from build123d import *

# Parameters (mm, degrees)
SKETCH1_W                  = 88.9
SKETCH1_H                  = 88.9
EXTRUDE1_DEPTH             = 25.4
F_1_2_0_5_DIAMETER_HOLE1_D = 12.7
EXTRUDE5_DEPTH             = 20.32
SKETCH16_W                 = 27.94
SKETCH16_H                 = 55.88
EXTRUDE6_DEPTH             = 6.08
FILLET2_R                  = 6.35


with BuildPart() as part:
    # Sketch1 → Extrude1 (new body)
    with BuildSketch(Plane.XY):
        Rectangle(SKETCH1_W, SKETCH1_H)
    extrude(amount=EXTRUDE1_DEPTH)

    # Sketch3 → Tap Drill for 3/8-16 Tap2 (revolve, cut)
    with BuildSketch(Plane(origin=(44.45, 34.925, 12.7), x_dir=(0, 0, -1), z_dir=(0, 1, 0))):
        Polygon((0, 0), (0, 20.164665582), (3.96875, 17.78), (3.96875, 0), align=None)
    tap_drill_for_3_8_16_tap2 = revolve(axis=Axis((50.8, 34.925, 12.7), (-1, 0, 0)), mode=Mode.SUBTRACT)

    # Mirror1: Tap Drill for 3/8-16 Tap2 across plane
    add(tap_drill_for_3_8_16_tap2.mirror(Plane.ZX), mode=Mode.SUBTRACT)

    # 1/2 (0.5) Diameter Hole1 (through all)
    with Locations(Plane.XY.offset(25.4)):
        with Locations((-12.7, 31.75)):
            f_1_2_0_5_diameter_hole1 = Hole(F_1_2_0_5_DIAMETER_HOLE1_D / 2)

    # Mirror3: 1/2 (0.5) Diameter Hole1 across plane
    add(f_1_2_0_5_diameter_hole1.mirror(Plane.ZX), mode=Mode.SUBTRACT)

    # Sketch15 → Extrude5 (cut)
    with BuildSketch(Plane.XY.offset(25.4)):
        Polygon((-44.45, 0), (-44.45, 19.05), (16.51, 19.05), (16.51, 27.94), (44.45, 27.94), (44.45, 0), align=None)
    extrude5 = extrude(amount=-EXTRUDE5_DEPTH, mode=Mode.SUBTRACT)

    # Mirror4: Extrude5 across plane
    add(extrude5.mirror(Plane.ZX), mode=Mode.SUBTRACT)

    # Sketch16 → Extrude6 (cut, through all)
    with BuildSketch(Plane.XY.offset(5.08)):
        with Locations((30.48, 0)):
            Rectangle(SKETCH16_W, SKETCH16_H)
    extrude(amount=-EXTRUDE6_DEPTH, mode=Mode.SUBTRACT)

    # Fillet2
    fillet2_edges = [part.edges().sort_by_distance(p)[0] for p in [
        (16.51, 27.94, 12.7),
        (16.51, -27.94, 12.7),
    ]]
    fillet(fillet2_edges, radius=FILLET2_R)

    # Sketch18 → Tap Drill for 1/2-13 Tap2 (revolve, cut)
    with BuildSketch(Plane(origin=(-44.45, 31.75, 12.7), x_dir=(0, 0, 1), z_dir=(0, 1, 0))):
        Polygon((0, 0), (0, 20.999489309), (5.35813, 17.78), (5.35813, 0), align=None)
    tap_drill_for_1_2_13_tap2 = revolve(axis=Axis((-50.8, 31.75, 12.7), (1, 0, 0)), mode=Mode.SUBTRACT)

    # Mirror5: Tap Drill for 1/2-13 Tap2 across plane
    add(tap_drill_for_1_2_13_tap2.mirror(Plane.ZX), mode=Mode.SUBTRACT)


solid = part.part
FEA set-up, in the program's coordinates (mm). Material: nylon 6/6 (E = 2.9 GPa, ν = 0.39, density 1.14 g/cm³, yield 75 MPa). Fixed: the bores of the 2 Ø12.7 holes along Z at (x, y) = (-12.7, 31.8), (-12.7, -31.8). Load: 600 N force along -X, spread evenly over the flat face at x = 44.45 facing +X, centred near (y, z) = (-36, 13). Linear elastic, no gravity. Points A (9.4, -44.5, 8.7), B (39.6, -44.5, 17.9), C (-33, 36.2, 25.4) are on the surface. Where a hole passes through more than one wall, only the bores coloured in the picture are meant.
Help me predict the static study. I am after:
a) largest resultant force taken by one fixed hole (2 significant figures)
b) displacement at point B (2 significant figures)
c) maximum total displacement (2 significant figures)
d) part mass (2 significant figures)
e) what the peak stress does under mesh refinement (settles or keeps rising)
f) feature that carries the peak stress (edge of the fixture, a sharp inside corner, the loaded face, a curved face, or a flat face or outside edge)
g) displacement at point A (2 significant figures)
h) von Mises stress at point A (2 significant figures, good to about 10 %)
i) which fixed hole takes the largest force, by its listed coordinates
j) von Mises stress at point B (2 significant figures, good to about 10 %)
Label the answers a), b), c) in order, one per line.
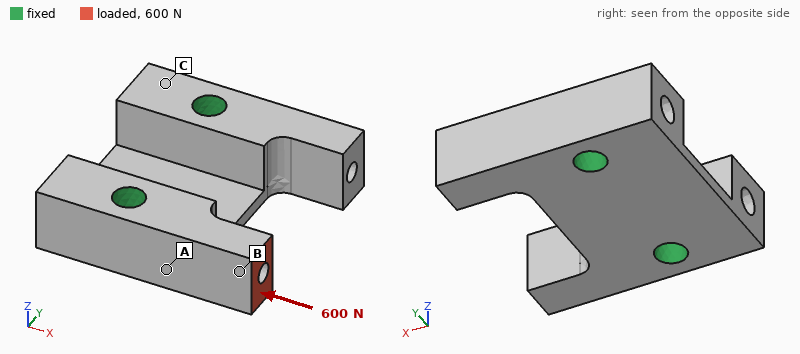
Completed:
a) 610 N
b) 43 µm
c) 48 µm
d) 120 g
e) keeps rising
f) edge of the fixture
g) 15 µm
h) 1.8 MPa
i) (-12.7, -31.8)
j) 1.6 MPa
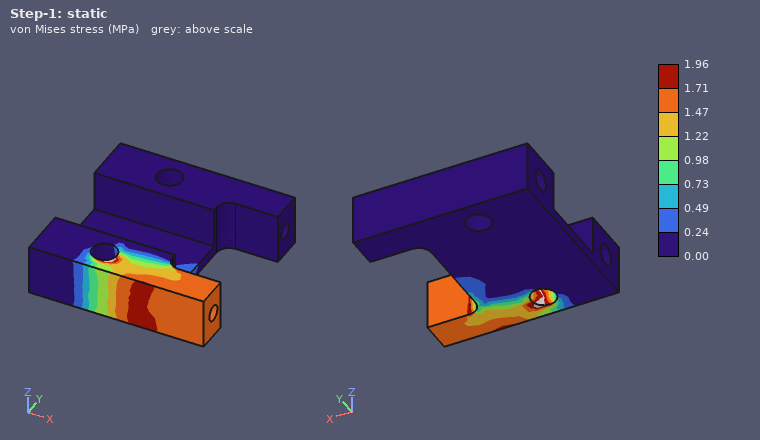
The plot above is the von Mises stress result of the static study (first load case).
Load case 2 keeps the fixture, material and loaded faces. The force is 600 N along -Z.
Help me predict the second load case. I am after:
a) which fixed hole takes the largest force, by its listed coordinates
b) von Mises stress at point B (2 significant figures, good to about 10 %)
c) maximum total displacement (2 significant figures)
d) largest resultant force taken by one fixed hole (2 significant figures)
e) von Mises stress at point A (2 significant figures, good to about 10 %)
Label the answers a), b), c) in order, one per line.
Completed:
a) (-12.7, -31.8)
b) 4.0 MPa
c) 0.46 mm
d) 610 N
e) 3.7 MPa
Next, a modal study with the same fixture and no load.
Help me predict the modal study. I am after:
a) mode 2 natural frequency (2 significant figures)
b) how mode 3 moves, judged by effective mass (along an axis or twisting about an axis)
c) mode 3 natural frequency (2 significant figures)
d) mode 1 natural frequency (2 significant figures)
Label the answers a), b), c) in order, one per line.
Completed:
a) 2300 Hz
b) along Z
c) 2400 Hz
d) 2300 Hz
